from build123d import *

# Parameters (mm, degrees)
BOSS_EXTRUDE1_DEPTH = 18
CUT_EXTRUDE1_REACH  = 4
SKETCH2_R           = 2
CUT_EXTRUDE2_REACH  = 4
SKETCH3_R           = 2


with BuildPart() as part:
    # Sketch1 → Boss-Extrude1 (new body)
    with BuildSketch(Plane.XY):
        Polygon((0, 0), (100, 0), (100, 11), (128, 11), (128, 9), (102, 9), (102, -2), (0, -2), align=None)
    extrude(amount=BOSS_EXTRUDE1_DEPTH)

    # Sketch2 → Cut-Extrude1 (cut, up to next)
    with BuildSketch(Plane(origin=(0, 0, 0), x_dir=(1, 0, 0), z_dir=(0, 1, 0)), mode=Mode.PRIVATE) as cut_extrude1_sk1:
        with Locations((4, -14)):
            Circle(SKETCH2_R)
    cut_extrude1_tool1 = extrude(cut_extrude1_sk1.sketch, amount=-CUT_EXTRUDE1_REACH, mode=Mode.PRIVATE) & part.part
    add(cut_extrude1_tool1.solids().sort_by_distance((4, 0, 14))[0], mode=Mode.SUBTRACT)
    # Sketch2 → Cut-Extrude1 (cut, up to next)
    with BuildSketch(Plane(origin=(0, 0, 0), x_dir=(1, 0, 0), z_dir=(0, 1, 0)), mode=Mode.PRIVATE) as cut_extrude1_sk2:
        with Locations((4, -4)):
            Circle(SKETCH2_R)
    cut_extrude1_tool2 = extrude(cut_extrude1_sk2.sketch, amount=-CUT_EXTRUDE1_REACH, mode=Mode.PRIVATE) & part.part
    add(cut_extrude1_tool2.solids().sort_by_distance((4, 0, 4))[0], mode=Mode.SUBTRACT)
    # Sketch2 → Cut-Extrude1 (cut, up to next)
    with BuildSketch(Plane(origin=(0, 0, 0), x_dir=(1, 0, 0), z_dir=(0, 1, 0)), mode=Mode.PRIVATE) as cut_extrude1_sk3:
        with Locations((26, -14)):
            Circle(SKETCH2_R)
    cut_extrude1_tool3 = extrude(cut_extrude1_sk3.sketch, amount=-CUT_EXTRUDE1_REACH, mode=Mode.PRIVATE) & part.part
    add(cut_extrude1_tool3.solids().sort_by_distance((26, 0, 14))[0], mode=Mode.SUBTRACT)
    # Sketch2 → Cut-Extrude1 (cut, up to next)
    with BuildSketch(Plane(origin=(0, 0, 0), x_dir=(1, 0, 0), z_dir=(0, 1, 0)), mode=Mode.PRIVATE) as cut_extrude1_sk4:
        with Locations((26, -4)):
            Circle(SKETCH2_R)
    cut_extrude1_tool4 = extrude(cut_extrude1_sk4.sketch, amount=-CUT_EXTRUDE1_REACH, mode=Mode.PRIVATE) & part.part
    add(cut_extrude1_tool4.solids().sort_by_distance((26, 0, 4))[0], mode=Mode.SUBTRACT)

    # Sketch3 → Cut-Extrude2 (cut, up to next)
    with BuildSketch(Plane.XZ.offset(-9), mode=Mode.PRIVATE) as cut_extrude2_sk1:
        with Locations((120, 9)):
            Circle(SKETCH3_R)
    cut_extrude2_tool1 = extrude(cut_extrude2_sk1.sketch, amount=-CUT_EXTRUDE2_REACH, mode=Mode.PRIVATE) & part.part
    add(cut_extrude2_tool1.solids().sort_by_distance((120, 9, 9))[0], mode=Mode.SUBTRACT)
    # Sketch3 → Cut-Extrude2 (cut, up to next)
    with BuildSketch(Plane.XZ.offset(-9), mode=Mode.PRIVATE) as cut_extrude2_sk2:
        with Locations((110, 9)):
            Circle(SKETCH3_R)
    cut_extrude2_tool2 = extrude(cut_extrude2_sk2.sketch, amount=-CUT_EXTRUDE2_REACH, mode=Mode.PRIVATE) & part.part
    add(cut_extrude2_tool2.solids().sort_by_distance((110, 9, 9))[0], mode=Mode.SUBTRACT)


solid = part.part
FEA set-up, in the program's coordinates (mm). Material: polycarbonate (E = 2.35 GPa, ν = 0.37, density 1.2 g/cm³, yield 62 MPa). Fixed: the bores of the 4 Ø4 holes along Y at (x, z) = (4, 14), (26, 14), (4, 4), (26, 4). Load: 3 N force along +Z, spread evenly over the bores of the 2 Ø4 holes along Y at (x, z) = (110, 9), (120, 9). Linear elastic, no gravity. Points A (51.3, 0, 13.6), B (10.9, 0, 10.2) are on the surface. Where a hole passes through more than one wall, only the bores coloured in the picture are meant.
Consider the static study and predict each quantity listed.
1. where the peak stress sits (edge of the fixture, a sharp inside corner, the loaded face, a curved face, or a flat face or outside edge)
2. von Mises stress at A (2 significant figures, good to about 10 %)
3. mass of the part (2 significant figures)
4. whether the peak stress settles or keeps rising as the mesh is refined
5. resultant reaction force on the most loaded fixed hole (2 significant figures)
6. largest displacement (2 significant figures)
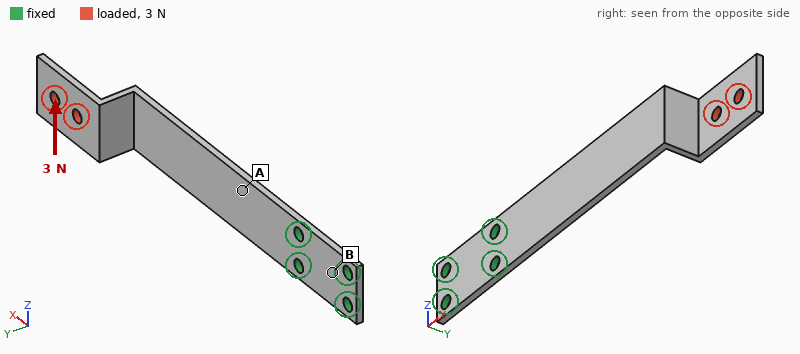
edge of the fixture
2.8 MPa
5.8 g
keeps rising
22 N
1.3 mm
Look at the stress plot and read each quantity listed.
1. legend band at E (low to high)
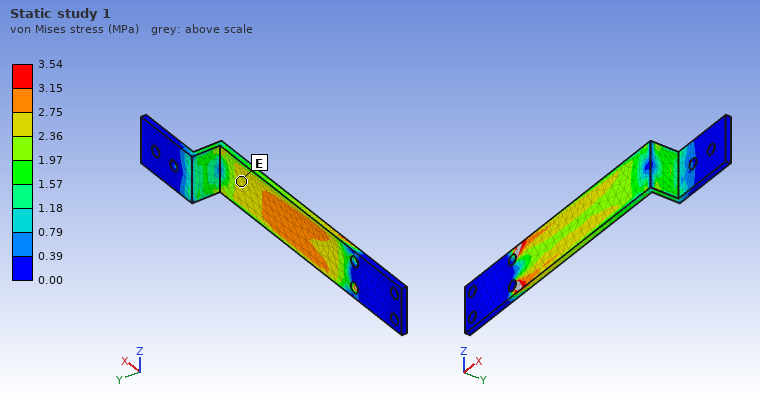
2.36 to 2.75 MPa
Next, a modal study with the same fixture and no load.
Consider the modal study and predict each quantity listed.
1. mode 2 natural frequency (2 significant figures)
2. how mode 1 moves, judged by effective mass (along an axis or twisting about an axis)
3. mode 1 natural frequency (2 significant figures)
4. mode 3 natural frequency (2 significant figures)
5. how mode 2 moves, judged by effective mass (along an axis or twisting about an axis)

220 Hz
along Y
42 Hz
250 Hz
along Z
